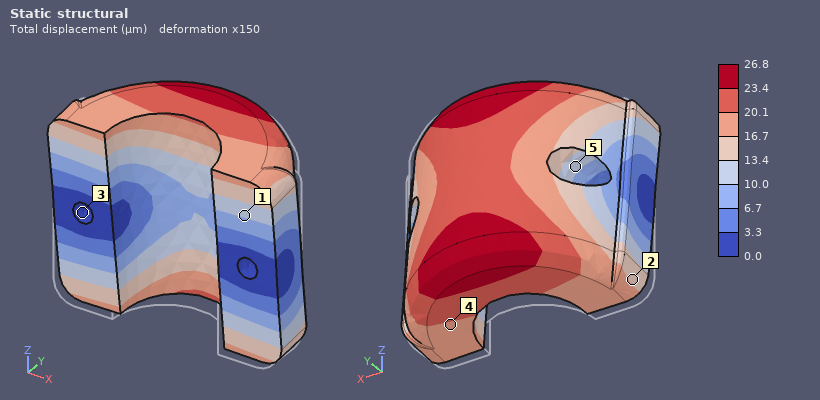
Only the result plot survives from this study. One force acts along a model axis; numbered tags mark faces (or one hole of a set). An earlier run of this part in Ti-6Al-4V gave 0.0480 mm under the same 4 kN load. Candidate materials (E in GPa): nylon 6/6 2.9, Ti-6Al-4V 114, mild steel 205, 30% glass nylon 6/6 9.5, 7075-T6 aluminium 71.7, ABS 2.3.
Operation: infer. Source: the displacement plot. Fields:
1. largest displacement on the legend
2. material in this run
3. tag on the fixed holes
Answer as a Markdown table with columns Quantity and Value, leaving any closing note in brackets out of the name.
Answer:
| Quantity | Value |
|---|---|
| largest displacement on the legend | 26.8 µm |
| material in this run | mild steel |
| tag on the fixed holes | 3 |
